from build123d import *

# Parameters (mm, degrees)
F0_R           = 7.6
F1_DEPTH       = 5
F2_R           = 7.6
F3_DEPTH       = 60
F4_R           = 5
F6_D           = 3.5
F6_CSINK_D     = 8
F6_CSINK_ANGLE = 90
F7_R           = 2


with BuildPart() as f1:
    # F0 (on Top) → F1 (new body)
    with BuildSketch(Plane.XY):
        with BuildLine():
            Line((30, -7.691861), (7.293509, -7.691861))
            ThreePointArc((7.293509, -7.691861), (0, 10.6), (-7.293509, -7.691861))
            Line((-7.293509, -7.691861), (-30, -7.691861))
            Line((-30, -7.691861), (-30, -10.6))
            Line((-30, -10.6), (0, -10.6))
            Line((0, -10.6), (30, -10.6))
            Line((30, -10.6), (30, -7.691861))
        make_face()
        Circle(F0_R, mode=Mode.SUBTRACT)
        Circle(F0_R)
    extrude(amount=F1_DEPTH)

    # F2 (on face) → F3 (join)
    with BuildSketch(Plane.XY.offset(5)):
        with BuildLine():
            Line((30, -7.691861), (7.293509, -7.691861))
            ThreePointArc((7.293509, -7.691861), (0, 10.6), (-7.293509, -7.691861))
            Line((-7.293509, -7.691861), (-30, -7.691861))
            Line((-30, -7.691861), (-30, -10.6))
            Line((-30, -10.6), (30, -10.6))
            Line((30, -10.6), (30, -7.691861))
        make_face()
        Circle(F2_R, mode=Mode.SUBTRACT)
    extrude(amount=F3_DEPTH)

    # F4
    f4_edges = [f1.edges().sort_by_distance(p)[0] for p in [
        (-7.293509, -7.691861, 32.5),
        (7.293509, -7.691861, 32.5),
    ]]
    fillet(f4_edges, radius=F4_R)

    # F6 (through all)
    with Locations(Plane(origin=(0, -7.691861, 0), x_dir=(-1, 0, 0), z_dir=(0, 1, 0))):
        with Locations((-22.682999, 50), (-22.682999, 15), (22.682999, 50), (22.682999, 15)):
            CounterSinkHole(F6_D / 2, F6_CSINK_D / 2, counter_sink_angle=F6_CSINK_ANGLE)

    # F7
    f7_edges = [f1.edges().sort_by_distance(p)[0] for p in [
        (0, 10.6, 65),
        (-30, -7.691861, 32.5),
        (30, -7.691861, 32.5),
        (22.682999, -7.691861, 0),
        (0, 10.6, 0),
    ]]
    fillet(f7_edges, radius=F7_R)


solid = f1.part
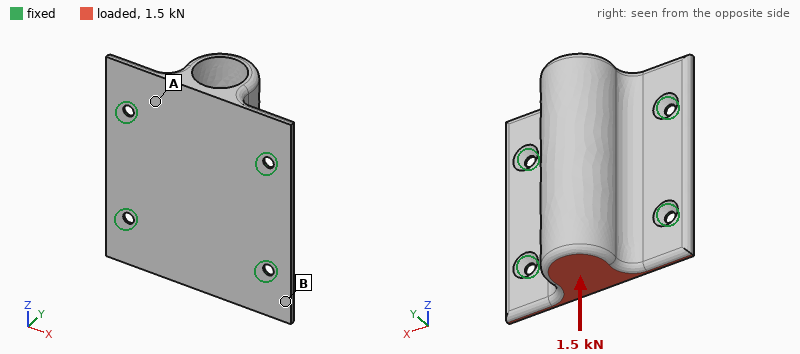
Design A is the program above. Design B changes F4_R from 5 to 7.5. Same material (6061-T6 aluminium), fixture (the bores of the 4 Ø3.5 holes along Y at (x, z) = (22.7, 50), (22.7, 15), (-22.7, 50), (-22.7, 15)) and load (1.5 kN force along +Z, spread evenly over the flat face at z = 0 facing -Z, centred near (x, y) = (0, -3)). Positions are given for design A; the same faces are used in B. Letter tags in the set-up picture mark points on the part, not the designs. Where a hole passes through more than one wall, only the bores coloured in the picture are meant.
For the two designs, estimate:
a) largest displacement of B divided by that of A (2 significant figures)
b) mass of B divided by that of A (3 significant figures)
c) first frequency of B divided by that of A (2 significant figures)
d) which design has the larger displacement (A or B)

0.74
1.05
1.1
A
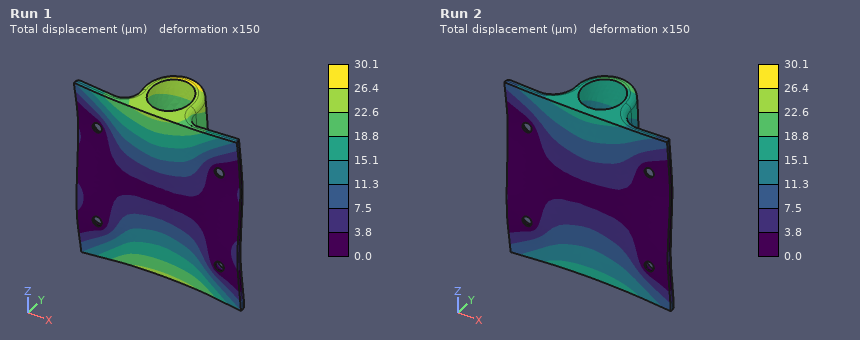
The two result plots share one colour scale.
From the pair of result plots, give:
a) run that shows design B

Run 2
